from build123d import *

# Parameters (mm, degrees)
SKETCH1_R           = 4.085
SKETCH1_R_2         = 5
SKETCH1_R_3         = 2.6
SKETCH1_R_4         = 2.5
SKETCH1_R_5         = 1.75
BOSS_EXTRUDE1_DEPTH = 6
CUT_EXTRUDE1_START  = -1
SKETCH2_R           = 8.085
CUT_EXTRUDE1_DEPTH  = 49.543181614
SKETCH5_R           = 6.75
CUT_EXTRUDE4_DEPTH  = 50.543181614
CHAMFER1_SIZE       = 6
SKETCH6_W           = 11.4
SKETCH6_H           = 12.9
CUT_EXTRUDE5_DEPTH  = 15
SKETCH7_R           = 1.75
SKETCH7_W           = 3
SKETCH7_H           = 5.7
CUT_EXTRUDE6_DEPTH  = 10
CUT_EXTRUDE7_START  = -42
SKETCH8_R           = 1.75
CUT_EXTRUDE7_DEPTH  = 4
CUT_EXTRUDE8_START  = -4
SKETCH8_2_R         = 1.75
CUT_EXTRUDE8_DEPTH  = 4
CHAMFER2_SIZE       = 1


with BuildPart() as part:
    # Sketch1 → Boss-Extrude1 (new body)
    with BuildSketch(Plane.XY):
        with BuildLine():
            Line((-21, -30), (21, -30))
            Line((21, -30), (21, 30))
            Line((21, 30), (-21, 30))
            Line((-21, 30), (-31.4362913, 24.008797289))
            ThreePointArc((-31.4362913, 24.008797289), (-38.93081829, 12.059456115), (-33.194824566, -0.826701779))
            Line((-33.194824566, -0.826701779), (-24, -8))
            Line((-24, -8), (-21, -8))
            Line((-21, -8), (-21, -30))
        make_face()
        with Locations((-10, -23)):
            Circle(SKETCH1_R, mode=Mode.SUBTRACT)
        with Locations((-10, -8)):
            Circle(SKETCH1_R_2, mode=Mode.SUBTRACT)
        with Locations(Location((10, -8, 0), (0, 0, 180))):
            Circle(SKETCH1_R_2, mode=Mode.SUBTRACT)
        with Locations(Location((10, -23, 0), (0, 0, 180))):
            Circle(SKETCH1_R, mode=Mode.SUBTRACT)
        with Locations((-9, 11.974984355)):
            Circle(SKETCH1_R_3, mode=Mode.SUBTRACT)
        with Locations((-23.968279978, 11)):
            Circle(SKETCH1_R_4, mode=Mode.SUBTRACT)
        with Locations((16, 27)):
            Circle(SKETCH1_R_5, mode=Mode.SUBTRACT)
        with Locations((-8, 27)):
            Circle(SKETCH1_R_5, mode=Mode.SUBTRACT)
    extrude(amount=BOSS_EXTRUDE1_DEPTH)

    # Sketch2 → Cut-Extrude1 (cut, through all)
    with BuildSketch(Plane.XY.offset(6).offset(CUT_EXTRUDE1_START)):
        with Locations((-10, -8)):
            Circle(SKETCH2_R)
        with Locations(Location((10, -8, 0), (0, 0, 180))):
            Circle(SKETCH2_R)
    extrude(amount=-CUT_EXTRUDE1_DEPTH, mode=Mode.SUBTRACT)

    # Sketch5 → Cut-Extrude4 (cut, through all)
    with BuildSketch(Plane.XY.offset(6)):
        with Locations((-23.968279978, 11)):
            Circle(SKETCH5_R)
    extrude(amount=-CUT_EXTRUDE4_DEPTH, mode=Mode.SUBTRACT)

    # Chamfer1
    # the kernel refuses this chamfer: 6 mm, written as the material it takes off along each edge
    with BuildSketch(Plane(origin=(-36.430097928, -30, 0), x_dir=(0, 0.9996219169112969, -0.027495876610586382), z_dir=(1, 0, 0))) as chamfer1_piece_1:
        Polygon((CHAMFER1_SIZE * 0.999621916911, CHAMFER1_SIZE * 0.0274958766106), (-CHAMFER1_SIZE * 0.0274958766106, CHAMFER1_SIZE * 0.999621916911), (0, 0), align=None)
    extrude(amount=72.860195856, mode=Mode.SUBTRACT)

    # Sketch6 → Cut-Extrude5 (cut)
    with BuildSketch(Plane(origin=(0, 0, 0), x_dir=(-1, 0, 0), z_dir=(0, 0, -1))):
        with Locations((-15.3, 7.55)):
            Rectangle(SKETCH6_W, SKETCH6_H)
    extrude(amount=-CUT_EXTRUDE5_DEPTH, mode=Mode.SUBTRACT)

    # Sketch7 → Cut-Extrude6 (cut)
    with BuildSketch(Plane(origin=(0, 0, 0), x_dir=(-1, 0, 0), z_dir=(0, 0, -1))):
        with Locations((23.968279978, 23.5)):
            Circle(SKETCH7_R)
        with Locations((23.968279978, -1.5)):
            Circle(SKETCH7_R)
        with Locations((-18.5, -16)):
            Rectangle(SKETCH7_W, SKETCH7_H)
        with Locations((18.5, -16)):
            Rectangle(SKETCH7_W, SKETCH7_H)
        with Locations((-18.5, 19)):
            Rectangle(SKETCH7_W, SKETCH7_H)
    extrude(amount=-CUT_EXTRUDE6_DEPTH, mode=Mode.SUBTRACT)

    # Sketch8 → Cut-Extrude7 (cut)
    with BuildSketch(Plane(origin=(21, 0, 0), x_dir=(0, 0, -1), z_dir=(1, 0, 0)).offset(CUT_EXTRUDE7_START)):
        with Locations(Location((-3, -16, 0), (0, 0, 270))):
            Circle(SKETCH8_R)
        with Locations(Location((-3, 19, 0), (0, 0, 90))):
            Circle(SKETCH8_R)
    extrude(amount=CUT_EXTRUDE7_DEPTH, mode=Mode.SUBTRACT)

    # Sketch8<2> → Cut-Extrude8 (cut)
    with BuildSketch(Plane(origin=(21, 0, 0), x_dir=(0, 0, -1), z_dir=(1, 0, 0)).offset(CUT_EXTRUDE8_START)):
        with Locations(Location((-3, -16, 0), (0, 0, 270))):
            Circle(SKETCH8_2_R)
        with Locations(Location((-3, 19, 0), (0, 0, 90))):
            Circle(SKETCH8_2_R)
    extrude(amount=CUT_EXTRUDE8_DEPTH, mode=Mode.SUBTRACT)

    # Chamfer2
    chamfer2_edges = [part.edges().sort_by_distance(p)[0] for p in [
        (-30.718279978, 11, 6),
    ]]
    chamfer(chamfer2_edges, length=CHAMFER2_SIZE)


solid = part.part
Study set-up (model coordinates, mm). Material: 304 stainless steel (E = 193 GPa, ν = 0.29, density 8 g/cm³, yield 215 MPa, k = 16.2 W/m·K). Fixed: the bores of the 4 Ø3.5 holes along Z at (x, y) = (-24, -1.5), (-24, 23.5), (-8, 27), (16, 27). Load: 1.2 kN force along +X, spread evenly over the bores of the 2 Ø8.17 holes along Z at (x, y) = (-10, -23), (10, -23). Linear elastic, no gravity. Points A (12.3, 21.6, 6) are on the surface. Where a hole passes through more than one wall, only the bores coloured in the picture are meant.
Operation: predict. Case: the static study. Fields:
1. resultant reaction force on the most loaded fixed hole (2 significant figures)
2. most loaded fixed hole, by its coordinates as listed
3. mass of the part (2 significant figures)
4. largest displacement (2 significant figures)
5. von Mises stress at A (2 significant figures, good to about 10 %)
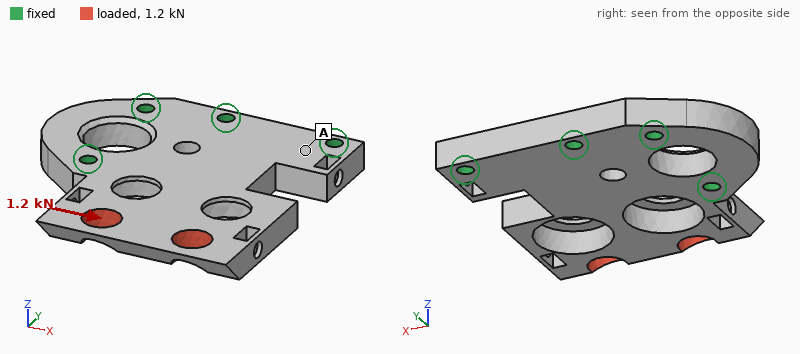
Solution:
1.4 kN
(-24, -1.5)
96 g
26 µm
14 MPa
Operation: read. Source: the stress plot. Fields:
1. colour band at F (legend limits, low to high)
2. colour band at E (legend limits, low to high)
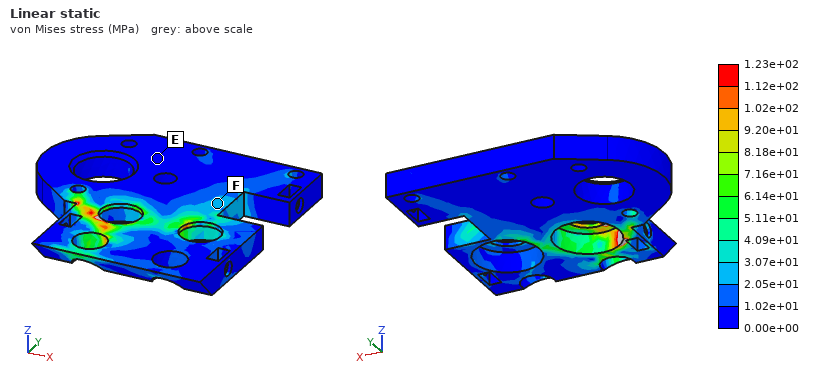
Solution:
2.05e+01 to 3.07e+01 MPa
0.00e+00 to 1.02e+01 MPa
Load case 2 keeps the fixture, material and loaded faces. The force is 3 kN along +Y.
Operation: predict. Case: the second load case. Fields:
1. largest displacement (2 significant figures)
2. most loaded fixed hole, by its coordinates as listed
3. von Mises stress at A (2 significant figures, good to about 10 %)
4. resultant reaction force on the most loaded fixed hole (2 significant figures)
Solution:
27 µm
(-8, 27)
25 MPa
1.6 kN
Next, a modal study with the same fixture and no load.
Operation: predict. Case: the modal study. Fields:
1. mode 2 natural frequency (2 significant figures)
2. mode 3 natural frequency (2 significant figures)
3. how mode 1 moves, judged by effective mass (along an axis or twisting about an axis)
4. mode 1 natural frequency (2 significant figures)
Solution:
5900 Hz
8600 Hz
along Z
2300 Hz
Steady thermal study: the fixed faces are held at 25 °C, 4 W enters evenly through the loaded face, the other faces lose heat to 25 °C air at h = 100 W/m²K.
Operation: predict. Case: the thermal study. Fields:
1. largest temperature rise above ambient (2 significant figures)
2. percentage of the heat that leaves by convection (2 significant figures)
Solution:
23 K
90 %
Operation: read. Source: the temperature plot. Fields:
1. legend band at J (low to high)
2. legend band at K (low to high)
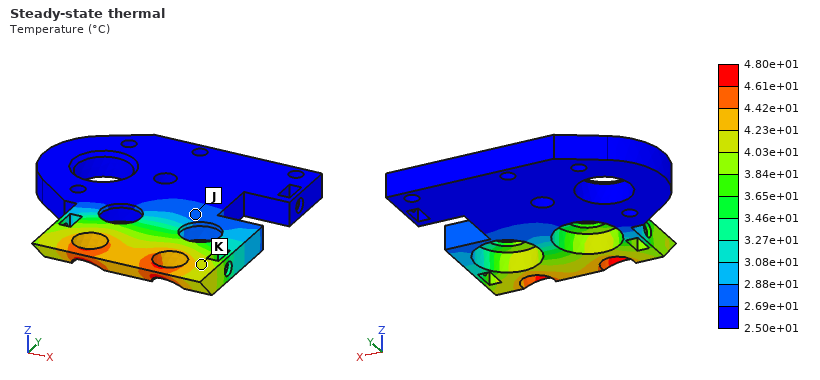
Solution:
2.69e+01 to 2.88e+01 °C
4.03e+01 to 4.23e+01 °C
